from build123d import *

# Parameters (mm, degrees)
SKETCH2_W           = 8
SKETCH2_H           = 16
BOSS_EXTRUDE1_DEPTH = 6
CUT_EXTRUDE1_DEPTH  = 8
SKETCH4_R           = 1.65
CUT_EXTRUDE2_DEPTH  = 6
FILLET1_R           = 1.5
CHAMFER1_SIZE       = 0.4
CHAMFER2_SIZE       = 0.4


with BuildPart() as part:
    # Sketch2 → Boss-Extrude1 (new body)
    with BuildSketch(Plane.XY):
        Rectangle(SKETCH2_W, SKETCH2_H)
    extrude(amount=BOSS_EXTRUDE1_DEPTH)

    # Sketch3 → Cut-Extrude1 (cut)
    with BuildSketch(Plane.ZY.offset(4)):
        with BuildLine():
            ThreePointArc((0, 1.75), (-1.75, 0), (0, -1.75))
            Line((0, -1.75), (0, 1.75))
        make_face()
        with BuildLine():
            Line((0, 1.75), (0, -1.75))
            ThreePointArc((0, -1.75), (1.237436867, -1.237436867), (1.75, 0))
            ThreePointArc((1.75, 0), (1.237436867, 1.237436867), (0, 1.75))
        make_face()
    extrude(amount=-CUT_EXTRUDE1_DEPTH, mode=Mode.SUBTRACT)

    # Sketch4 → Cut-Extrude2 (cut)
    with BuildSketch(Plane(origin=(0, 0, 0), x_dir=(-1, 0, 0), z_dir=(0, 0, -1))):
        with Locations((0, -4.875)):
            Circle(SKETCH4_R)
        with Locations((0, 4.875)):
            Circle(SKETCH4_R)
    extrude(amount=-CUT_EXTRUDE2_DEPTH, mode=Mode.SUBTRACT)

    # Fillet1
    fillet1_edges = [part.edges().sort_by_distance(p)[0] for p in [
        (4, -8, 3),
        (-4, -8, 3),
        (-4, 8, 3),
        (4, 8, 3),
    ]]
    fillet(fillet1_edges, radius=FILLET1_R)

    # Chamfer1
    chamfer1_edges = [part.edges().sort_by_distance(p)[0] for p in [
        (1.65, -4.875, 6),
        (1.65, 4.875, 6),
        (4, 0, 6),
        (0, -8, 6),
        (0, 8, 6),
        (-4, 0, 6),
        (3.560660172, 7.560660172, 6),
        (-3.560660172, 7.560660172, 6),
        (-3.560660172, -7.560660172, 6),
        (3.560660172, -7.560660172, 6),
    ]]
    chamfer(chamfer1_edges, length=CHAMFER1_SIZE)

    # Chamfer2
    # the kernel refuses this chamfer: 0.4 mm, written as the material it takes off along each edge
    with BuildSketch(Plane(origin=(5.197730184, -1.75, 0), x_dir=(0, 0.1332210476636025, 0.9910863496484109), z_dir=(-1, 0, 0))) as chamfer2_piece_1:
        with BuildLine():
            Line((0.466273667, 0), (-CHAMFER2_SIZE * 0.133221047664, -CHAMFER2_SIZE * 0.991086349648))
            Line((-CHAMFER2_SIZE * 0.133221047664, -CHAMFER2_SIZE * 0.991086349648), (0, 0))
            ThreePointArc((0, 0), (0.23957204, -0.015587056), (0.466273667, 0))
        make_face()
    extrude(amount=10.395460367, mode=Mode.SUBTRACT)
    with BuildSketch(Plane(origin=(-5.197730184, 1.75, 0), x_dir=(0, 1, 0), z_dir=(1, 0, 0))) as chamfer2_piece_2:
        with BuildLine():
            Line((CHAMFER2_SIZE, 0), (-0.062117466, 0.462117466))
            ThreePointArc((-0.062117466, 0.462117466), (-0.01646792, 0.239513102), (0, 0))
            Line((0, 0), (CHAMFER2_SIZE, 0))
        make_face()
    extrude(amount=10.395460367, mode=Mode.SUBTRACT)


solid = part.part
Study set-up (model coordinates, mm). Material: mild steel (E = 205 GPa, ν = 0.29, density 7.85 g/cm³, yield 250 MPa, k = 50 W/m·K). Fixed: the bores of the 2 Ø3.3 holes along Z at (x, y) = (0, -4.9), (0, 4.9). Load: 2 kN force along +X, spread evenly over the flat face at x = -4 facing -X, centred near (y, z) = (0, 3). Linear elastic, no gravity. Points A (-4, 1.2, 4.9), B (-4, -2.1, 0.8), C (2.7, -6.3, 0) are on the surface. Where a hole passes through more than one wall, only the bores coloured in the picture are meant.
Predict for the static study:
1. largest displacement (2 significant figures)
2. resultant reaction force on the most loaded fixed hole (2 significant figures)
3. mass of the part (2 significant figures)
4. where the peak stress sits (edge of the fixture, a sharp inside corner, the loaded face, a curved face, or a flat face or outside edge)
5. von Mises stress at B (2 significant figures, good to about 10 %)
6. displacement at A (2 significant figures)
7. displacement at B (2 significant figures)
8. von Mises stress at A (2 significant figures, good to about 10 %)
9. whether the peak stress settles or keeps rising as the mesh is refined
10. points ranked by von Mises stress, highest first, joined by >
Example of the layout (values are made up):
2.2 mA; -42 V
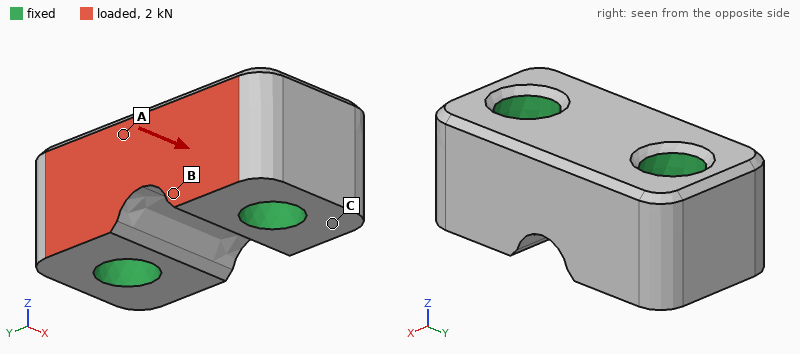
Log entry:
0.75 µm; 1.0 kN; 4.8 g; edge of the fixture; 28 MPa; 0.70 µm; 0.70 µm; 19 MPa; keeps rising; B > A > C
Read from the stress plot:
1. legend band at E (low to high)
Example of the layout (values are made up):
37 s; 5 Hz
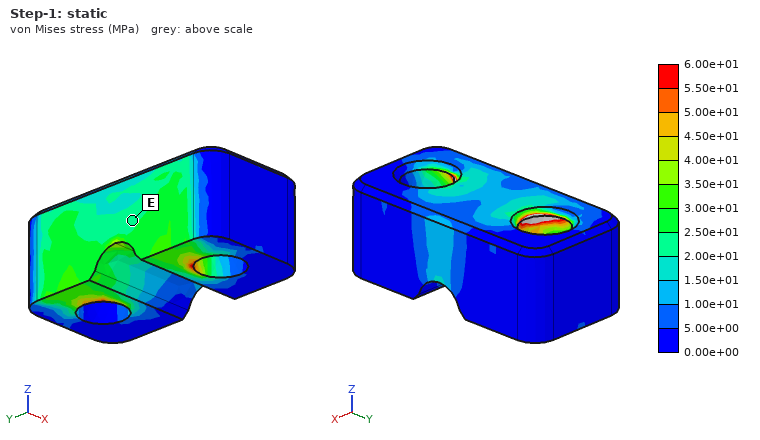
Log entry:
2.00e+01 to 2.50e+01 MPa
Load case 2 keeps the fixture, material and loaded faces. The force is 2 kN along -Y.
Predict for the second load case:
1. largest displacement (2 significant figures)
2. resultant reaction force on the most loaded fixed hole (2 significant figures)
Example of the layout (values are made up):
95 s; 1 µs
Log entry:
1.6 µm; 1.1 kN
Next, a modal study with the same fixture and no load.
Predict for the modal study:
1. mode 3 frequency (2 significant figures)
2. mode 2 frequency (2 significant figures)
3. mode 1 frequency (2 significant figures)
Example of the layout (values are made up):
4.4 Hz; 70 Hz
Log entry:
190 kHz; 170 kHz; 160 kHz
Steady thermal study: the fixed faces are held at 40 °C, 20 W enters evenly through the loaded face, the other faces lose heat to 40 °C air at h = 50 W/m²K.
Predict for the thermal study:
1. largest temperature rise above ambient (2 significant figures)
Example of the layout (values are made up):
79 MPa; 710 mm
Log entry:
20 K
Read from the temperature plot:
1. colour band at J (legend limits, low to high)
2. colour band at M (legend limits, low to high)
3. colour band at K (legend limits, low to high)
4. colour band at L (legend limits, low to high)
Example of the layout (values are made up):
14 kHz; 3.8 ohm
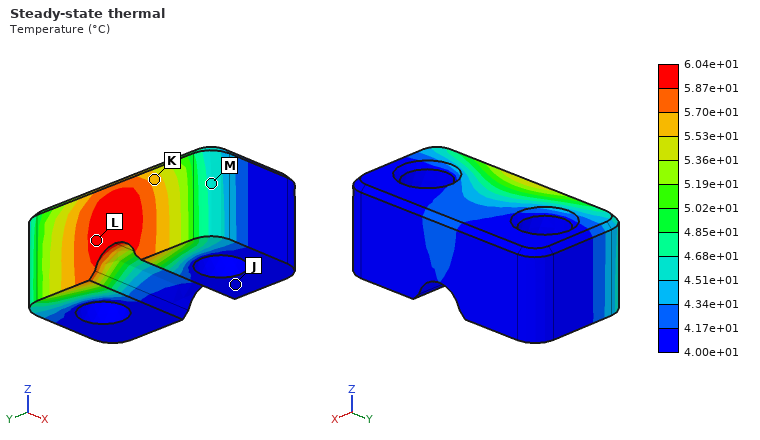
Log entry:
4.00e+01 to 4.17e+01 °C; 4.51e+01 to 4.68e+01 °C; 5.53e+01 to 5.70e+01 °C; 5.87e+01 to 6.04e+01 °C
